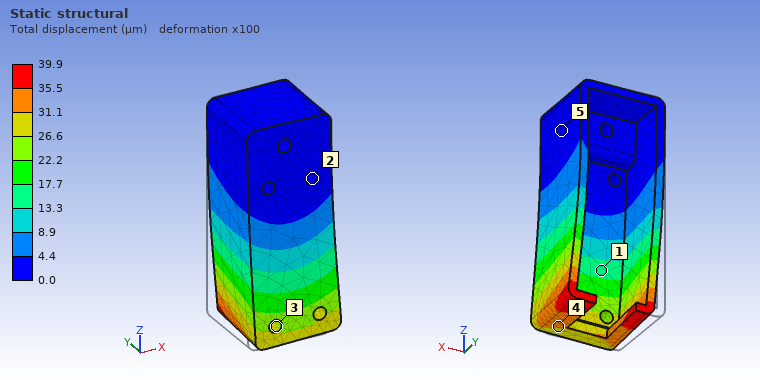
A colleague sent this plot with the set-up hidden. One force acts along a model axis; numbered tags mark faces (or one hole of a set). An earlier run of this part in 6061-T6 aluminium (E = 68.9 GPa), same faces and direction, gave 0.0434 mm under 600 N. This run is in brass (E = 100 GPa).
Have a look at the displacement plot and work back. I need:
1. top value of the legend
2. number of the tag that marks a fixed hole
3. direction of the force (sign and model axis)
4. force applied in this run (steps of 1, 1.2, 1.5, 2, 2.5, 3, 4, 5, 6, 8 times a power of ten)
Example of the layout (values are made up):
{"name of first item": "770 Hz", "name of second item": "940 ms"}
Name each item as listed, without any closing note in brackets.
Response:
{"top value of the legend": "39.9 µm", "number of the tag that marks a fixed hole": "2", "direction of the force": "+X", "force applied in this run": "800 N"}
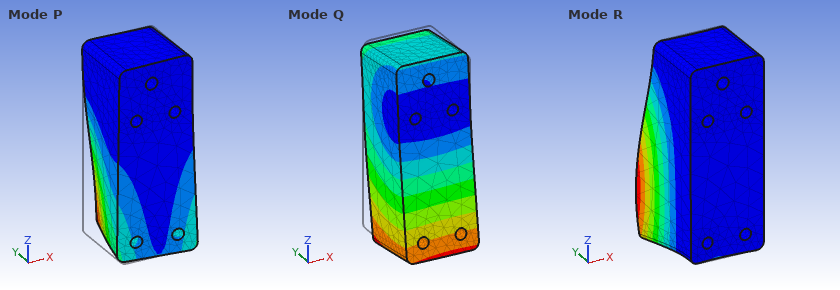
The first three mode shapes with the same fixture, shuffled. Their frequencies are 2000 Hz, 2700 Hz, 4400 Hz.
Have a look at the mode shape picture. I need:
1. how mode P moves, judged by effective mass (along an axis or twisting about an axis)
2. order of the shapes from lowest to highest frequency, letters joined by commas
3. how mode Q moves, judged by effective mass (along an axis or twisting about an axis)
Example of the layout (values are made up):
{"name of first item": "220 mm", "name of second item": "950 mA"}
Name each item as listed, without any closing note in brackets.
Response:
{"how mode P moves, judged by effective mass": "along X", "order of the shapes from lowest to highest frequency, letters joined by commas": "Q, P, R", "how mode Q moves, judged by effective mass": "along Y"}
